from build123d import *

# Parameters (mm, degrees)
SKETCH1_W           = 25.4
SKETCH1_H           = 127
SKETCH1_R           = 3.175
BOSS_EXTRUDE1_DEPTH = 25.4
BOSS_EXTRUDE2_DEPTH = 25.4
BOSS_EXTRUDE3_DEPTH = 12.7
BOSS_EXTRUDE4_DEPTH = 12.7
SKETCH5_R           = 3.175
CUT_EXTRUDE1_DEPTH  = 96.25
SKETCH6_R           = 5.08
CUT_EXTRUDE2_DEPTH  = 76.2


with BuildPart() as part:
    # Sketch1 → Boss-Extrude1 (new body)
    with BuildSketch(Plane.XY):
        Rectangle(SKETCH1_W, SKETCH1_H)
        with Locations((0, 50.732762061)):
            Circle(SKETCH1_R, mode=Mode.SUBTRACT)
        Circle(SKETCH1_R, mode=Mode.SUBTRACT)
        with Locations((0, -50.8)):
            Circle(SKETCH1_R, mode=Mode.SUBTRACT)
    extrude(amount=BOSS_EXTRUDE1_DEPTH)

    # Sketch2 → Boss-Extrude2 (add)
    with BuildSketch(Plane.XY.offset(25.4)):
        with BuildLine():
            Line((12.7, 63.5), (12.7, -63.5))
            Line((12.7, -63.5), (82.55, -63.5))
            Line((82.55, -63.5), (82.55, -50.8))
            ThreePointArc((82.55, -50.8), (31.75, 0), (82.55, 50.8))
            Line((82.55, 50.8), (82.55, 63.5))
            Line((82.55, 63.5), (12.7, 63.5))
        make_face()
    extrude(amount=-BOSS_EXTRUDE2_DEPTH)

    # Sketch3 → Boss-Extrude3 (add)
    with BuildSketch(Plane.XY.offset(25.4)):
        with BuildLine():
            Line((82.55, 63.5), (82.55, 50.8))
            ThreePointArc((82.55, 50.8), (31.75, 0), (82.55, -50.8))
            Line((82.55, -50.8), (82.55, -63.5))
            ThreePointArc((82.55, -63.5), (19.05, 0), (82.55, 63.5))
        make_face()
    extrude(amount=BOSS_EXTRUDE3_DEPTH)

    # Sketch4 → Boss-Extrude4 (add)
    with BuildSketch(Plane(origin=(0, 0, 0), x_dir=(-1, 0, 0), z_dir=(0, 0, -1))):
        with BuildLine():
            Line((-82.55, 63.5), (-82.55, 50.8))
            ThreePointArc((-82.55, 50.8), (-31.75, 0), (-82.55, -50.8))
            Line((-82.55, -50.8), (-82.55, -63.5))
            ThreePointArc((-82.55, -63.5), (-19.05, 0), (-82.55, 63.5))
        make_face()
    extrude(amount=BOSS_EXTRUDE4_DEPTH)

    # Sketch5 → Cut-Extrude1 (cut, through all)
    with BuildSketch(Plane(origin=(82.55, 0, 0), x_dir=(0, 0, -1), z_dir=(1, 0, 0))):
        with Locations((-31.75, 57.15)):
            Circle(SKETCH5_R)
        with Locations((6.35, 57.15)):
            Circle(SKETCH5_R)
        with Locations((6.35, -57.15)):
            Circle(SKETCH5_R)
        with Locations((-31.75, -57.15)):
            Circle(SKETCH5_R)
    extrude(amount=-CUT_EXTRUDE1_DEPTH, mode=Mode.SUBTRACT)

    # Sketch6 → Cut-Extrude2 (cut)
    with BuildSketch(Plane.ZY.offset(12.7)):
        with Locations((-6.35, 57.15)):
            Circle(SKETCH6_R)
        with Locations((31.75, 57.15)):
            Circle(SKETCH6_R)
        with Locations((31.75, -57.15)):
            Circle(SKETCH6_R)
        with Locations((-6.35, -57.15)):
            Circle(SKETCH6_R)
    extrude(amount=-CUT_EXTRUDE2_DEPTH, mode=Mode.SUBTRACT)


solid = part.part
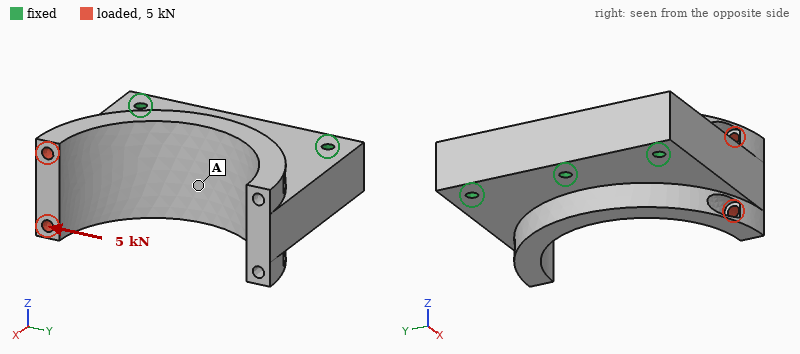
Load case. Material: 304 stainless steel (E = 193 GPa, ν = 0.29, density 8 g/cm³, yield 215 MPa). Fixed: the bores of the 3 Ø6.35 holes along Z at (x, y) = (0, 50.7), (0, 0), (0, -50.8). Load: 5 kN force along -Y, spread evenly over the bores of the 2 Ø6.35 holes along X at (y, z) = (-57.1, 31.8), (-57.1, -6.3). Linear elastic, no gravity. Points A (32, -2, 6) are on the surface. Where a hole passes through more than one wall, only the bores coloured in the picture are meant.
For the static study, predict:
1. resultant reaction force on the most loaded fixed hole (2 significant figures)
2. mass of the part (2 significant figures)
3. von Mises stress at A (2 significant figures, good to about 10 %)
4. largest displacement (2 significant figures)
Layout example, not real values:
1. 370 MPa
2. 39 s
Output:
1. 5.7 kN
2. 2.0 kg
3. 7.9 MPa
4. 38 µm
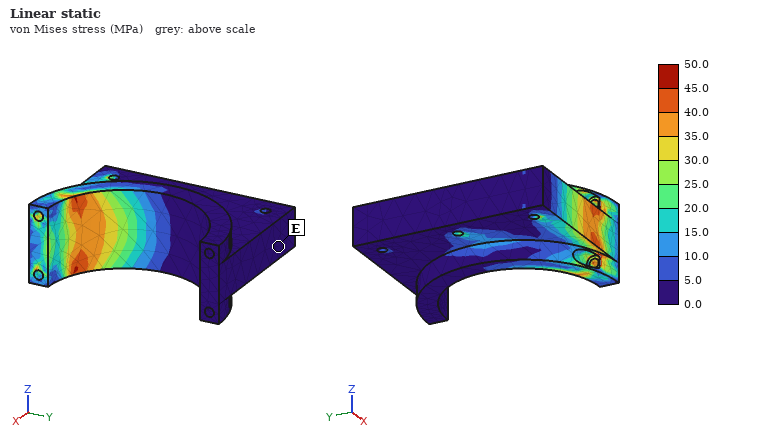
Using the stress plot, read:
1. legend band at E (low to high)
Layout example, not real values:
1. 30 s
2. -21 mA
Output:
1. 0.0 to 5.0 MPa
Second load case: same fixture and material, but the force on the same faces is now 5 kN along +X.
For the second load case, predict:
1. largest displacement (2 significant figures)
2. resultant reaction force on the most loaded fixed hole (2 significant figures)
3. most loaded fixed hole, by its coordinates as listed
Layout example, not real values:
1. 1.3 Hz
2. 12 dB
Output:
1. 14 µm
2. 5.3 kN
3. (0, -50.8)
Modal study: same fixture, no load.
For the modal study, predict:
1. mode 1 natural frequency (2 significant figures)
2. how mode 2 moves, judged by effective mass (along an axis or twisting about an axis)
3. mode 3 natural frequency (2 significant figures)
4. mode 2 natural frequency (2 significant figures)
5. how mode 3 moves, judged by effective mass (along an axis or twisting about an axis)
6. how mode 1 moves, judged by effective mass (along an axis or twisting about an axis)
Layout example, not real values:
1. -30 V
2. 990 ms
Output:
1. 3100 Hz
2. twisting about X
3. 6000 Hz
4. 3500 Hz
5. along Y
6. along Z
